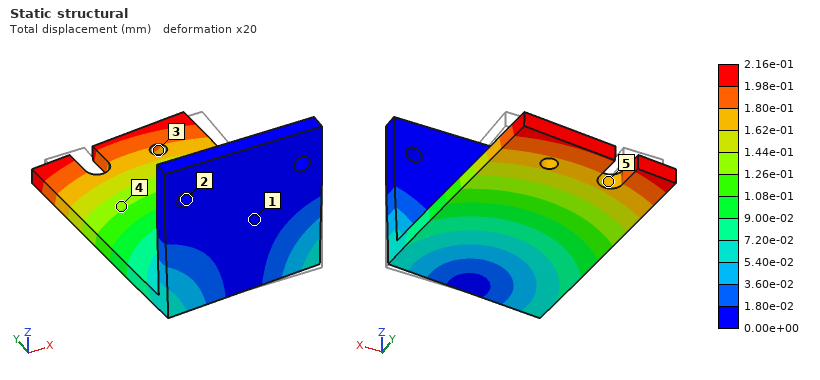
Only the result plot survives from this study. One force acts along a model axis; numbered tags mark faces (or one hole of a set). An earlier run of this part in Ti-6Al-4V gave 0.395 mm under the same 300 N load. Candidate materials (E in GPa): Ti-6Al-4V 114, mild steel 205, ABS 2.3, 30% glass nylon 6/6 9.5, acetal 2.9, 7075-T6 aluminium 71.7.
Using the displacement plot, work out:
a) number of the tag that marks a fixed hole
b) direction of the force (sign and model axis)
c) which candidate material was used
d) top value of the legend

2
-X
mild steel
2.16e-01 mm
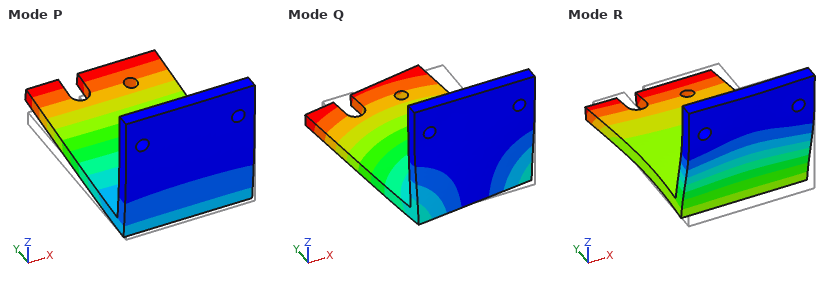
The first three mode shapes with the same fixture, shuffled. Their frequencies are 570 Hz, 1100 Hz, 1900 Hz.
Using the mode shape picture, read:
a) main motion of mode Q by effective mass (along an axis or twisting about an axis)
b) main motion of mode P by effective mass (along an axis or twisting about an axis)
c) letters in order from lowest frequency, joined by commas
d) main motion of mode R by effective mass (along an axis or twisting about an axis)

along X
along Z
P, Q, R
along Y
